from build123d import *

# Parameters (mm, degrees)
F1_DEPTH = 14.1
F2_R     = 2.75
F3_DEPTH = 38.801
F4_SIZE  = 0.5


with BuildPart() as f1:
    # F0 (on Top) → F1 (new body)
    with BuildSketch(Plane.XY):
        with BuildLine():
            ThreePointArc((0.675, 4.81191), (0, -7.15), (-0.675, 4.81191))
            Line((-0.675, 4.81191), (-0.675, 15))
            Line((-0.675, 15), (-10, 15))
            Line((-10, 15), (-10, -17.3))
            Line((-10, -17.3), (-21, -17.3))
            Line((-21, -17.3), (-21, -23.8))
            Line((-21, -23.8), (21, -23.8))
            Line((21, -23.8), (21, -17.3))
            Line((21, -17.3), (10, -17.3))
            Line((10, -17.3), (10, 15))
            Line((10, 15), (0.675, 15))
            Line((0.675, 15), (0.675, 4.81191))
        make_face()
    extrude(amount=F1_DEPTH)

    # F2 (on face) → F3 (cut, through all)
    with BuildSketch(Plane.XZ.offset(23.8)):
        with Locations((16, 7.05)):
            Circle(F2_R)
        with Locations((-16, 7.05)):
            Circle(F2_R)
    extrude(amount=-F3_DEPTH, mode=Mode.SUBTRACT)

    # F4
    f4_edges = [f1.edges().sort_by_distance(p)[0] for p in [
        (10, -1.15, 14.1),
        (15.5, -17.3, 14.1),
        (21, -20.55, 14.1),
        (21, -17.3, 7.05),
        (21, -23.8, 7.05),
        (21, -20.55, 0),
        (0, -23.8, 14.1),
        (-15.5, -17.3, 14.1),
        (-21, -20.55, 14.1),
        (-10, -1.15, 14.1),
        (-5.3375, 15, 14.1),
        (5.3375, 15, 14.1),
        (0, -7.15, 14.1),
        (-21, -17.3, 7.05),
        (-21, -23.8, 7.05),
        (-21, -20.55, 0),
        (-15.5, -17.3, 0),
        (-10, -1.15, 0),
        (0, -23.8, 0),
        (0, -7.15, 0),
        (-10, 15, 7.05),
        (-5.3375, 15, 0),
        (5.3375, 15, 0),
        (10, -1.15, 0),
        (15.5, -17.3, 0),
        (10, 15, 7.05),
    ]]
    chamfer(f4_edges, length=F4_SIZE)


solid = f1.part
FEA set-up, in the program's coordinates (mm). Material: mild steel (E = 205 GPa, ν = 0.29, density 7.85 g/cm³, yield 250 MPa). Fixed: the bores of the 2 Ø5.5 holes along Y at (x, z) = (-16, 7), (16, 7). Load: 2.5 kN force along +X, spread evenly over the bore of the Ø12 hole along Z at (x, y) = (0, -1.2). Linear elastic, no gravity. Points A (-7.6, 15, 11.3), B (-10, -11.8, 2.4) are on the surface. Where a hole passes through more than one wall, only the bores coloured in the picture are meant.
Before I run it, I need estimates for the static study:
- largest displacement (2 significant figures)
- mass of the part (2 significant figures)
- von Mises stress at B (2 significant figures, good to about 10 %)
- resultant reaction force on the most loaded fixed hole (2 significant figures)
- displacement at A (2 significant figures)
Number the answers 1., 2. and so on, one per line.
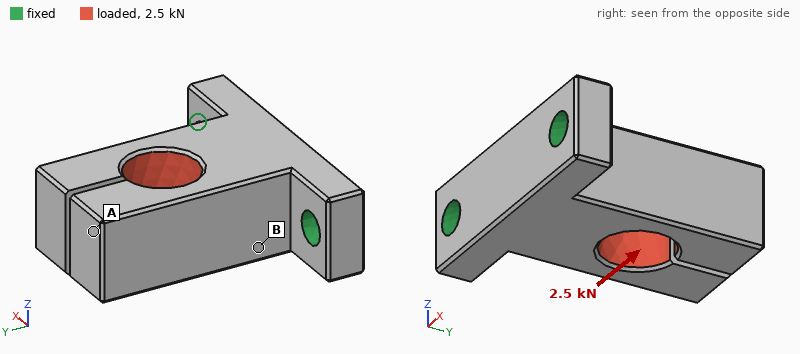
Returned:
1. 46 µm
2. 85 g
3. 42 MPa
4. 2.3 kN
5. 45 µm
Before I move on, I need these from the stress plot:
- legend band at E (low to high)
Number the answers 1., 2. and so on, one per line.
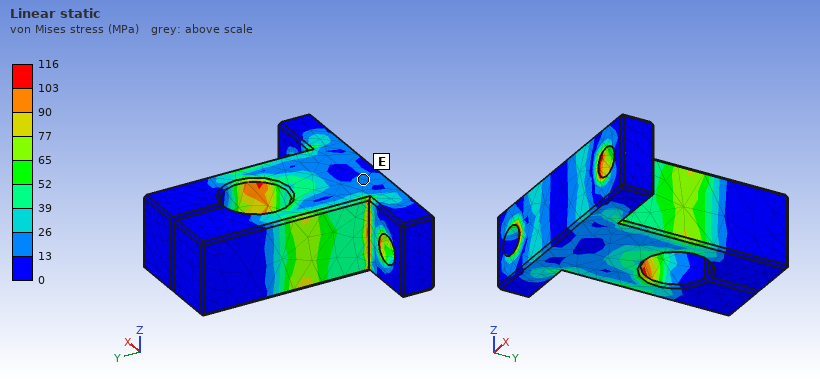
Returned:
1. 13 to 26 MPa
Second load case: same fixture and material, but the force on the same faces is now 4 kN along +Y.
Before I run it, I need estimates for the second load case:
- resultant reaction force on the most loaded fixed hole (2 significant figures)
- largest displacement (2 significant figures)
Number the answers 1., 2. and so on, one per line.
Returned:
1. 2.1 kN
2. 38 µm
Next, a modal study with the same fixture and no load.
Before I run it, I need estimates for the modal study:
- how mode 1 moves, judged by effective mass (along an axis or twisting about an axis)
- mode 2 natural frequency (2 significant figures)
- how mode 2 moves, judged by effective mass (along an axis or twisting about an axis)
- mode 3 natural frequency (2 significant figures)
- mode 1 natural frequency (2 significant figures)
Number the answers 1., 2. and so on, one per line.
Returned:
1. along Z
2. 4600 Hz
3. along X
4. 4900 Hz
5. 4200 Hz
